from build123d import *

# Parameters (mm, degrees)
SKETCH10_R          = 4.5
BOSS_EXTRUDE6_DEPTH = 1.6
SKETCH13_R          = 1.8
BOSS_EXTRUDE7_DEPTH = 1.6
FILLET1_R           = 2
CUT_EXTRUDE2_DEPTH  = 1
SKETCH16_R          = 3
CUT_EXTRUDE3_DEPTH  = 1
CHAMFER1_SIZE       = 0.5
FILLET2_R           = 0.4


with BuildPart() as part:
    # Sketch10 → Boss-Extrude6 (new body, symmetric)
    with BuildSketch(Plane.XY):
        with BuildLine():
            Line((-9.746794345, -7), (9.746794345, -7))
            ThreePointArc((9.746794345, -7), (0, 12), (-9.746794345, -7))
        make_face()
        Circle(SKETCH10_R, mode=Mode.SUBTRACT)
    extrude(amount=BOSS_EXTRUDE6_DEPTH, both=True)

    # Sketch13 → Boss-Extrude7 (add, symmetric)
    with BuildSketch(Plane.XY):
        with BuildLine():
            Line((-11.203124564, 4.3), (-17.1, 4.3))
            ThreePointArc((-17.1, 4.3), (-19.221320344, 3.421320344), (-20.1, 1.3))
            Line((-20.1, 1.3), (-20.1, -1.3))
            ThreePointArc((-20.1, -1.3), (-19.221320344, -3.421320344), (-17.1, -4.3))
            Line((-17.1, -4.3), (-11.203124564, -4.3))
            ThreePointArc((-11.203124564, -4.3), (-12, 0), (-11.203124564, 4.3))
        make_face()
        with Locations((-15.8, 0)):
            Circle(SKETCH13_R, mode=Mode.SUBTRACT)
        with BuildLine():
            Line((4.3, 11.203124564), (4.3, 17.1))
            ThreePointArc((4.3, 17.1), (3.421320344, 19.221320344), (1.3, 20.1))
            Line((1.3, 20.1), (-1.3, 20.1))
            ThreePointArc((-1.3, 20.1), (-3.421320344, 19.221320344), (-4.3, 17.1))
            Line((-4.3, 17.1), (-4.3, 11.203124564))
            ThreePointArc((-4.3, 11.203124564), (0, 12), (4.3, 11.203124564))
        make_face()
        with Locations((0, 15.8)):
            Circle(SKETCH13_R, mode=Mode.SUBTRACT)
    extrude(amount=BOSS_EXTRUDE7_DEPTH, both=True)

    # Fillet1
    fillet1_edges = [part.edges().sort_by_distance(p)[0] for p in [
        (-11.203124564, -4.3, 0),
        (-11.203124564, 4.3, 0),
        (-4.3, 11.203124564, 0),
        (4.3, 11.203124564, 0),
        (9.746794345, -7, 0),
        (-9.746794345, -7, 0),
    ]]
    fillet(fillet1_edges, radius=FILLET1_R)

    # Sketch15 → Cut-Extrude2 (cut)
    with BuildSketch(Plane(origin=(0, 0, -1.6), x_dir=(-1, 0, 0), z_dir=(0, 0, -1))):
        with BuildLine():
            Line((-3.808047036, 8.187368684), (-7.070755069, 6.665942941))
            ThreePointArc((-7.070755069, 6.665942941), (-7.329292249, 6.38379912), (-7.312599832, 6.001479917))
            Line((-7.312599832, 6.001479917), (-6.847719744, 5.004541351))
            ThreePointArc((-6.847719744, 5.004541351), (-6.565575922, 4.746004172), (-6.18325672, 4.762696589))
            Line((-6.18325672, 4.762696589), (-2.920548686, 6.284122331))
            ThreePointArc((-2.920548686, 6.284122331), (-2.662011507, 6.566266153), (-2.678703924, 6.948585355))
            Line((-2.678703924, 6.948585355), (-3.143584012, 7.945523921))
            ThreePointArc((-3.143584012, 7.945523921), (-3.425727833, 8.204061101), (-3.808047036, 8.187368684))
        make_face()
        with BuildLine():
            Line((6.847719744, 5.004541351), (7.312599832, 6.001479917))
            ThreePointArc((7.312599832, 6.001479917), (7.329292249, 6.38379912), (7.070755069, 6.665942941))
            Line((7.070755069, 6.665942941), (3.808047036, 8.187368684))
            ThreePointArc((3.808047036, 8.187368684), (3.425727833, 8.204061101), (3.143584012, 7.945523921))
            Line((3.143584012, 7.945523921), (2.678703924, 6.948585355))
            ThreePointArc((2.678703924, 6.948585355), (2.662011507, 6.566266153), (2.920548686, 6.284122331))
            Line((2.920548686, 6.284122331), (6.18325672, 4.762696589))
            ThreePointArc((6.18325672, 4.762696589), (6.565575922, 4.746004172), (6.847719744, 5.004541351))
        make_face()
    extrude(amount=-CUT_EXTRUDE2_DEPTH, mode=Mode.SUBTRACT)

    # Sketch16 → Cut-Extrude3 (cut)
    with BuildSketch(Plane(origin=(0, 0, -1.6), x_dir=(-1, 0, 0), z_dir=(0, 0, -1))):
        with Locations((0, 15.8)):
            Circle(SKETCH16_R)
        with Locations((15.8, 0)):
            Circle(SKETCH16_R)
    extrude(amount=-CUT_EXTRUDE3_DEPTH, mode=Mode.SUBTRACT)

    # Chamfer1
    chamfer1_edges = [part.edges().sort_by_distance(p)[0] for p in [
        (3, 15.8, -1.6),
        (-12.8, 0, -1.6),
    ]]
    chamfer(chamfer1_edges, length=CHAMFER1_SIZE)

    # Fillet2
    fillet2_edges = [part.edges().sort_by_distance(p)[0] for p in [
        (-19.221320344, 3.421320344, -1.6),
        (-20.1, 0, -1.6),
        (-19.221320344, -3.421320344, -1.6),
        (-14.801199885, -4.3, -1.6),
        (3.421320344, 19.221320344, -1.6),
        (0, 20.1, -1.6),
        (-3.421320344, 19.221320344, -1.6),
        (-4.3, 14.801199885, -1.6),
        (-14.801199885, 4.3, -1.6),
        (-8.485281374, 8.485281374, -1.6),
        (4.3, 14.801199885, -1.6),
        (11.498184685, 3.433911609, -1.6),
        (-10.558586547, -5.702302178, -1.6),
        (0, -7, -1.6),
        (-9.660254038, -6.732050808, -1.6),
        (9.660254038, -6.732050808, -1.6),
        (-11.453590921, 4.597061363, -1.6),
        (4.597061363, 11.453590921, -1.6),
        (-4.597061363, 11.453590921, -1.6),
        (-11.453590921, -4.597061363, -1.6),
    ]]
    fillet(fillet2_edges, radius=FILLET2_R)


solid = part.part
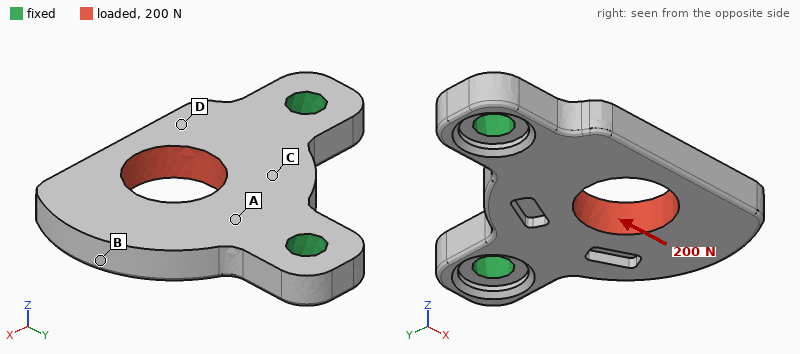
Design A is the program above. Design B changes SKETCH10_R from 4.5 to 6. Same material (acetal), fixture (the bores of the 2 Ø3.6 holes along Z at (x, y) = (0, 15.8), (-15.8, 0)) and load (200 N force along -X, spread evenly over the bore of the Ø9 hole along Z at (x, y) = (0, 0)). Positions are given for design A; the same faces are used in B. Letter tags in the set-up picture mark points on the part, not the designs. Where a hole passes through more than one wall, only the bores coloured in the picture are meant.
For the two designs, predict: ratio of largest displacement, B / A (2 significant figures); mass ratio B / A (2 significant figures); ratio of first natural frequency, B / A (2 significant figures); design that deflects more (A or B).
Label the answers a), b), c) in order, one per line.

a) 1.6
b) 0.88
c) 1.0
d) B
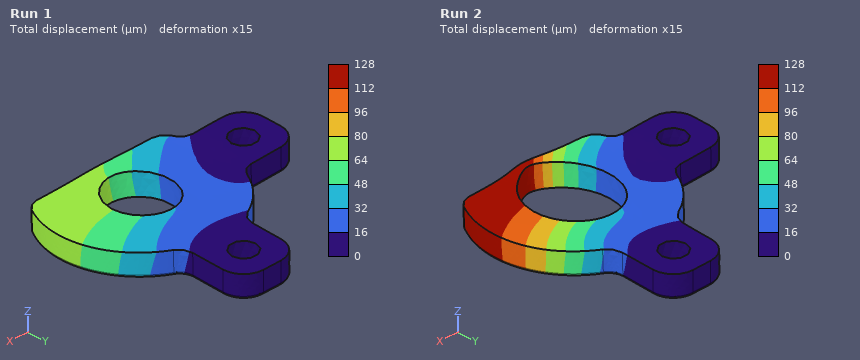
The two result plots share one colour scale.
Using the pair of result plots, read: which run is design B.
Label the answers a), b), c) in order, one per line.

a) Run 2
